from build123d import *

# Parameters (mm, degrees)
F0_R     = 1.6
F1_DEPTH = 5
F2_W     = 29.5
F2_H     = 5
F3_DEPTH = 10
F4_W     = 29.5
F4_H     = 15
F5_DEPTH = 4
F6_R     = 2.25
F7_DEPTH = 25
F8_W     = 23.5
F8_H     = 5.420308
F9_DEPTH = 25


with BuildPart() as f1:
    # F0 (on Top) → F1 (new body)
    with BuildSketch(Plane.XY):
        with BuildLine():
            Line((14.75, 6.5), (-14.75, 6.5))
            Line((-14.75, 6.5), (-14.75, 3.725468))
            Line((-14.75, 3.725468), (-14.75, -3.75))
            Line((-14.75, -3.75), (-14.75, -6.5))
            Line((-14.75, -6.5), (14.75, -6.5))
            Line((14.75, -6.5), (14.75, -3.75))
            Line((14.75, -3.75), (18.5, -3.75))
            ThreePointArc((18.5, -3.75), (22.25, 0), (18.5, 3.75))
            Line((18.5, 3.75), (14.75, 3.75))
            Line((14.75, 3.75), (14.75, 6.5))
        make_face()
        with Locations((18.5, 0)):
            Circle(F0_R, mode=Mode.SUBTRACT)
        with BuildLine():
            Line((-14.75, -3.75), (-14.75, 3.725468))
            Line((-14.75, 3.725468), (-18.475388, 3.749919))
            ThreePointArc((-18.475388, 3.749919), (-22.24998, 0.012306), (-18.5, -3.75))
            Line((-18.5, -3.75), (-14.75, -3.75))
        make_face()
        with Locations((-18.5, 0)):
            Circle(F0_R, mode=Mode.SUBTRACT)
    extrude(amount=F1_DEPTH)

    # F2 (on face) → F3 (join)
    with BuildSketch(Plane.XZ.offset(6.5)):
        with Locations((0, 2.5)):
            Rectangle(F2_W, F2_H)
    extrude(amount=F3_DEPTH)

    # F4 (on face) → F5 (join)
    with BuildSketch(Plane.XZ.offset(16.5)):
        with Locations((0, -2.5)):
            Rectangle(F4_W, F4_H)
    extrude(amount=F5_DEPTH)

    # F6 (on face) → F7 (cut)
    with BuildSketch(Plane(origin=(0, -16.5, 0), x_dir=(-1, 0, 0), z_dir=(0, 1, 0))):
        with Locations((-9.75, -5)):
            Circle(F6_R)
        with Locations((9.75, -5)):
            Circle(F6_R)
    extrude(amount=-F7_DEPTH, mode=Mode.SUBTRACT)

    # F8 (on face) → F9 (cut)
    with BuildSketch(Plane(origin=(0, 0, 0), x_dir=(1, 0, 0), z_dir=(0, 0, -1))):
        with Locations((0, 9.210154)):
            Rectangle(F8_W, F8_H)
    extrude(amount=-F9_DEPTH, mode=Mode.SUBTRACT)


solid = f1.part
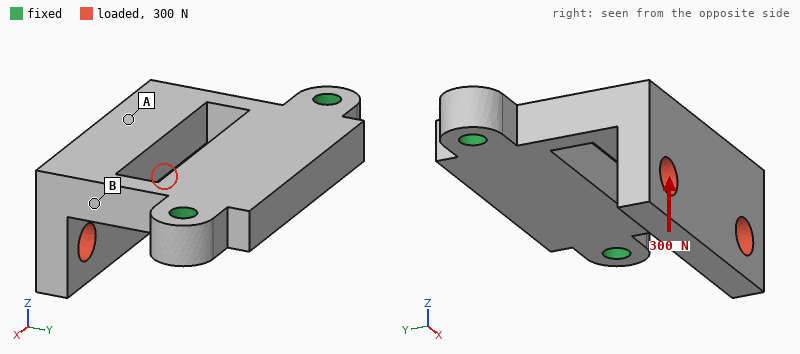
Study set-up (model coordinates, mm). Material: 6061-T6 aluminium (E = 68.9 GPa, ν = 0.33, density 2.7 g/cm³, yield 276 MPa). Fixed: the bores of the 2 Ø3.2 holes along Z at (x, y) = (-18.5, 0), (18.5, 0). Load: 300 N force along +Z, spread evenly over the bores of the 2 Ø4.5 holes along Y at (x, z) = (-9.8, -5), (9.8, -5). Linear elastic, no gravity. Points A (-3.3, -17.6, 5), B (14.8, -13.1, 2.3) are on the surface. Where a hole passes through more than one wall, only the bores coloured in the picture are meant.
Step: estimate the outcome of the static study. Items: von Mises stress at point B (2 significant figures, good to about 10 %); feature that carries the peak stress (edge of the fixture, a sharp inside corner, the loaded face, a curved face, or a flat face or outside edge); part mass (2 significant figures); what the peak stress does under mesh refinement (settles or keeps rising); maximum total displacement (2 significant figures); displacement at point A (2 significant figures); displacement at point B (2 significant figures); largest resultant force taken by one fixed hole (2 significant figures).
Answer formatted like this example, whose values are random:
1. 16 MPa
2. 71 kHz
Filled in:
1. 37 MPa
2. edge of the fixture
3. 13 g
4. keeps rising
5. 0.20 mm
6. 0.13 mm
7. 0.077 mm
8. 150 N
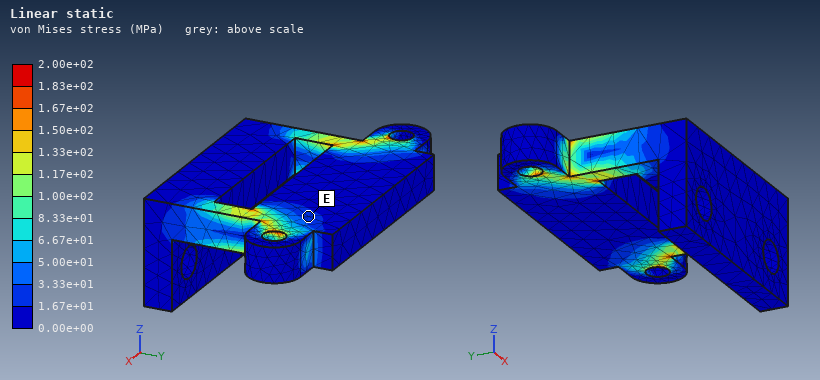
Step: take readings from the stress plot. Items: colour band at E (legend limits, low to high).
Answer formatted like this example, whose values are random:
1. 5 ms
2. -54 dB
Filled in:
1. 1.67e+01 to 3.33e+01 MPa
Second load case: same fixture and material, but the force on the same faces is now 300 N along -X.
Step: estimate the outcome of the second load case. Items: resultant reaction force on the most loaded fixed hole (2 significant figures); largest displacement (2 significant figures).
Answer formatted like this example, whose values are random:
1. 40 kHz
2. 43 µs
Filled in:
1. 230 N
2. 41 µm
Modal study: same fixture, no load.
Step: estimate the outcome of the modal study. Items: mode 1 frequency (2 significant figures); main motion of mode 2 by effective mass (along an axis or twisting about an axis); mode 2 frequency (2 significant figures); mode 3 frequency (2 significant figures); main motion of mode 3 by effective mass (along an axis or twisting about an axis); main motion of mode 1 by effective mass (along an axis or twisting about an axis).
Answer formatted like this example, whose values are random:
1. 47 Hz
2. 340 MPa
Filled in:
1. 2900 Hz
2. along X
3. 7100 Hz
4. 10 kHz
5. along X
6. along Z
